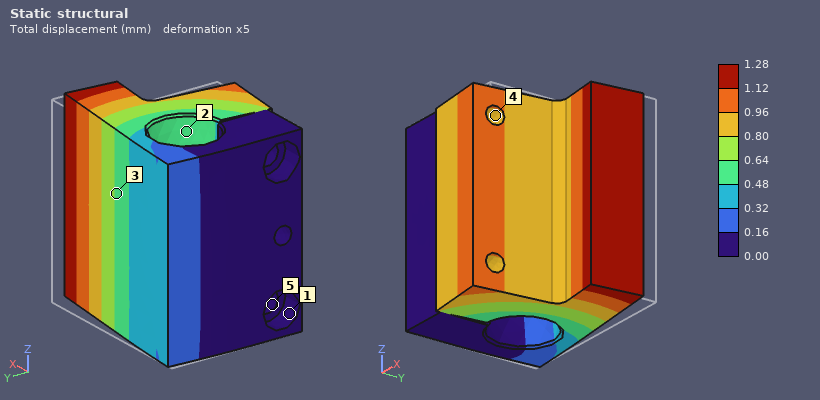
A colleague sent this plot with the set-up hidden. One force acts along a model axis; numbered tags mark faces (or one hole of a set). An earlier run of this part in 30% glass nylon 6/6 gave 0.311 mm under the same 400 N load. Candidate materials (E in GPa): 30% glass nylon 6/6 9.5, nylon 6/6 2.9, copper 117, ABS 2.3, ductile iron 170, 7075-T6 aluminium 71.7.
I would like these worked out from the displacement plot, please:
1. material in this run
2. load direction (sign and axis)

ABS
-Y
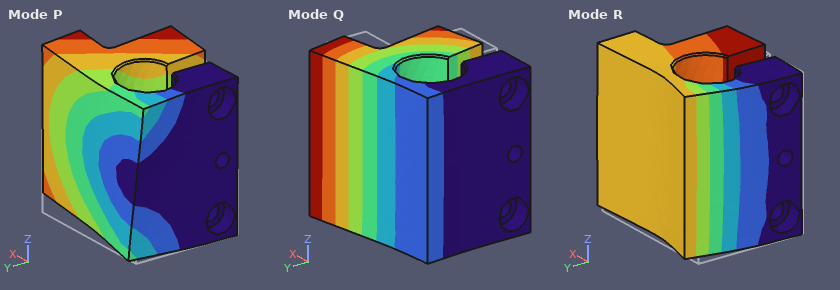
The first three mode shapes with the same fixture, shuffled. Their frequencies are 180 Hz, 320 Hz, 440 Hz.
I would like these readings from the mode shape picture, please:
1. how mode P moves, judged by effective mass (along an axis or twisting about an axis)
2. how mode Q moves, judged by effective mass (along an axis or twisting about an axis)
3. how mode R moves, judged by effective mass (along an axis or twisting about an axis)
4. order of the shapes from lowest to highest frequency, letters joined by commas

along Z
along Y
along X
Q, P, R
